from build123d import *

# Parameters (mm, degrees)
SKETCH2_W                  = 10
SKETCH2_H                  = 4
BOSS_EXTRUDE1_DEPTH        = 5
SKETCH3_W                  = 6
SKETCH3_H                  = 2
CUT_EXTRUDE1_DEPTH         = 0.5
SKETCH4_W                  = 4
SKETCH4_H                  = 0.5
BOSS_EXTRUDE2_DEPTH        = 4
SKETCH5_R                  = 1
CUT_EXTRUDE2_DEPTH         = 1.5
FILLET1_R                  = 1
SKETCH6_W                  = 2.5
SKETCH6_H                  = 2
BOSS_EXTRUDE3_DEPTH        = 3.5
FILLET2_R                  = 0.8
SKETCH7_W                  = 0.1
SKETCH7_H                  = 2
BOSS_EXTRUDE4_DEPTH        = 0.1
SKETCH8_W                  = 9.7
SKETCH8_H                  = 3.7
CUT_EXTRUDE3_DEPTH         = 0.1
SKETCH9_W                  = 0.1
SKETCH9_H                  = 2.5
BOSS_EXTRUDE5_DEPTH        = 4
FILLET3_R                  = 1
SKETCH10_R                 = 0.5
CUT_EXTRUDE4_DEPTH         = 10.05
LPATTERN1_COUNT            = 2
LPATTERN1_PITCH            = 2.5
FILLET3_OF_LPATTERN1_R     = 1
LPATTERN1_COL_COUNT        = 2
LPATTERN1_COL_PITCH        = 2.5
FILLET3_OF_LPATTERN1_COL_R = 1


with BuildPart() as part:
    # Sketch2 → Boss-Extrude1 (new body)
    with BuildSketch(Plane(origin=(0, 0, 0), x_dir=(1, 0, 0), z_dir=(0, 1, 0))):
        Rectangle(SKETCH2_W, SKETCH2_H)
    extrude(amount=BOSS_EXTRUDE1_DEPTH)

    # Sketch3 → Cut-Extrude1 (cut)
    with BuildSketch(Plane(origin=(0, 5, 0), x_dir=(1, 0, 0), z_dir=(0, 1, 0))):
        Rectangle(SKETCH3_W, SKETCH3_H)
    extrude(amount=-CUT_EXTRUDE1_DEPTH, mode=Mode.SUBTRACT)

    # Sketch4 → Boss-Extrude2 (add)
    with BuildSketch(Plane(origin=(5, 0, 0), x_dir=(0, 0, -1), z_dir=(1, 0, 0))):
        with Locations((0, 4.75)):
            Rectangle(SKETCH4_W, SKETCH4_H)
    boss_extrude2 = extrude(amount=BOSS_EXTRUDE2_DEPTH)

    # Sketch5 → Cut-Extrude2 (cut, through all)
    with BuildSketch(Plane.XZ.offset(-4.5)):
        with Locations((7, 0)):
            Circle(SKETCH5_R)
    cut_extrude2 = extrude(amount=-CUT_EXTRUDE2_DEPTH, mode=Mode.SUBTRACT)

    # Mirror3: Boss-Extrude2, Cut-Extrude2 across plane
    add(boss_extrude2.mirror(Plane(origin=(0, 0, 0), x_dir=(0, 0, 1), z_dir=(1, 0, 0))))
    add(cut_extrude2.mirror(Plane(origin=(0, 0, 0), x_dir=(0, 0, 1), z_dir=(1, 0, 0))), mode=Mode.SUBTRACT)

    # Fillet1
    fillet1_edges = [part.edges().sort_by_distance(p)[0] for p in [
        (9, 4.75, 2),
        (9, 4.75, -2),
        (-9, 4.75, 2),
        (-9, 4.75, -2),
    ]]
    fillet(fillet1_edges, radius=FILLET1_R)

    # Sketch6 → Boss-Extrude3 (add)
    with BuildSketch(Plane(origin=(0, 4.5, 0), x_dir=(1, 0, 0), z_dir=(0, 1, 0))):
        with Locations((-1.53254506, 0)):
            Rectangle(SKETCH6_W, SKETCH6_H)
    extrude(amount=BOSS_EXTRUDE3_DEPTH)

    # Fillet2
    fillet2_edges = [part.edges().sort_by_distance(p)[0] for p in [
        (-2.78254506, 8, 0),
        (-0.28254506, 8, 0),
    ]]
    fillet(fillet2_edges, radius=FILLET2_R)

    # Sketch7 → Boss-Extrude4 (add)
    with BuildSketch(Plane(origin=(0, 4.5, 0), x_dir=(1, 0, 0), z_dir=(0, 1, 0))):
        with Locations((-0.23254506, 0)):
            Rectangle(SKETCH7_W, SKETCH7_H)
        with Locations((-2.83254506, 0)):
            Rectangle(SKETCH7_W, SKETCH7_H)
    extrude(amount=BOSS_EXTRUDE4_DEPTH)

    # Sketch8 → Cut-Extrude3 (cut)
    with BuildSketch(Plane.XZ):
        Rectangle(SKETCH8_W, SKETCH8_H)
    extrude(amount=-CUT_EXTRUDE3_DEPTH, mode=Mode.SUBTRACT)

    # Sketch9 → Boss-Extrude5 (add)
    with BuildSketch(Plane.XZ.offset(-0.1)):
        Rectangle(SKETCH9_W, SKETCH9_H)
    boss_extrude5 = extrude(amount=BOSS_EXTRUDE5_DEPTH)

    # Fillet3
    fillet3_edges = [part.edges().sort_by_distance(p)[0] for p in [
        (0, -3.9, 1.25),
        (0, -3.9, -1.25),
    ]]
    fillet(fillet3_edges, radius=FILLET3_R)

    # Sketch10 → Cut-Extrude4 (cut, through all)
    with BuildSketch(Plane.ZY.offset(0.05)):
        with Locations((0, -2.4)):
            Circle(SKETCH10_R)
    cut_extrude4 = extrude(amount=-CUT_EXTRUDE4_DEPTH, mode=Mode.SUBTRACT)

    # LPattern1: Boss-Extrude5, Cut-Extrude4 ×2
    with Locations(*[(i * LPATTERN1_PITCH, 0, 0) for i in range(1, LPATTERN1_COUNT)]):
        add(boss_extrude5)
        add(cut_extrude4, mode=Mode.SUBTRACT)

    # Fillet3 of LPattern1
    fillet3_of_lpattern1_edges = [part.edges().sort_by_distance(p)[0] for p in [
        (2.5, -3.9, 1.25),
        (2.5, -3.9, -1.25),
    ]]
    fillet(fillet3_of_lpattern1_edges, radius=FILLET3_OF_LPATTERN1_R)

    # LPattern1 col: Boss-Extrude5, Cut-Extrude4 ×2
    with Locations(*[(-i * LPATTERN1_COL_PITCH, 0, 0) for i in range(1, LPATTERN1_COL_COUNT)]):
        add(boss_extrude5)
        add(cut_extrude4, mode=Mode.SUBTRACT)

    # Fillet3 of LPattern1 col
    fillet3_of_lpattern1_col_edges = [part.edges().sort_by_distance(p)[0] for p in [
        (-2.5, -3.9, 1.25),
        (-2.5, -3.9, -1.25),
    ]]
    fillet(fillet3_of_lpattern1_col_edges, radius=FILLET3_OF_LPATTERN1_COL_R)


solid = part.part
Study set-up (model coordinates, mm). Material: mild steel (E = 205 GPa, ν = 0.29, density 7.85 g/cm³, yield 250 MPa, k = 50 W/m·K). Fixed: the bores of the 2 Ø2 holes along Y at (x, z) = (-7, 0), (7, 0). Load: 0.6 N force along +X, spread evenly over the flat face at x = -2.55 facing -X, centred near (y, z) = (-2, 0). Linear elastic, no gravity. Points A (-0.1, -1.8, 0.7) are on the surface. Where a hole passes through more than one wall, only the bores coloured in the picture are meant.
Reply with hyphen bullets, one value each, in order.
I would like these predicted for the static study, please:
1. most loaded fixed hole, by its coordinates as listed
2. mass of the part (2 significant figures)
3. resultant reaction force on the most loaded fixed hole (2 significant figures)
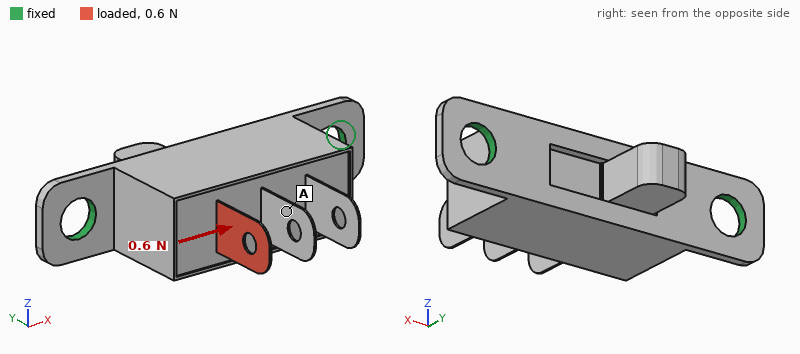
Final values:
- (7, 0)
- 1.7 g
- 0.51 N
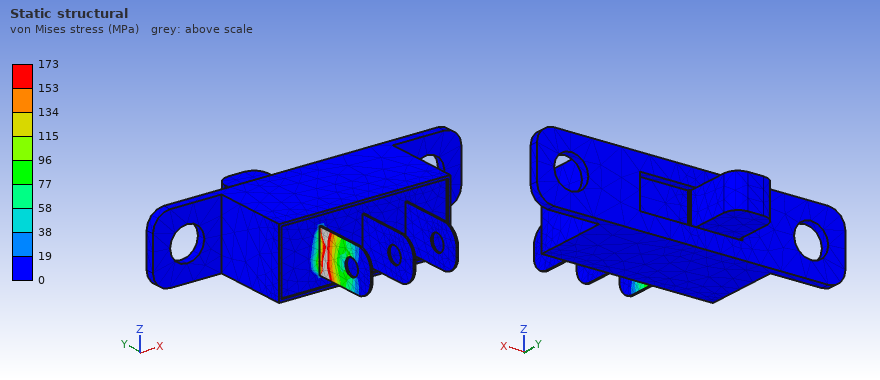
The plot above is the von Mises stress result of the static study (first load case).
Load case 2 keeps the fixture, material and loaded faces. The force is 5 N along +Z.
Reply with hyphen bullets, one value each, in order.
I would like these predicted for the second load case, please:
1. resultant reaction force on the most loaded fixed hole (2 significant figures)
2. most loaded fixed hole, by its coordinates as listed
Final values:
- 3.5 N
- (-7, 0)
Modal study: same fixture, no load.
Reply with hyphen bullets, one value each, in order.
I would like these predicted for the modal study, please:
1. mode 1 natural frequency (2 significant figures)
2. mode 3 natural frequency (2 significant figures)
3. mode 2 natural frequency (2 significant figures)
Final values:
- 5800 Hz
- 5900 Hz
- 5800 Hz
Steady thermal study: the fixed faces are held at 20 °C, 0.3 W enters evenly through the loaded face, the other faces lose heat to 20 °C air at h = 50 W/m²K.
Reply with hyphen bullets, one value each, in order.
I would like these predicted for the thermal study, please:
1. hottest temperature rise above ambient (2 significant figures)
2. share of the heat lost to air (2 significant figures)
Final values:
- 53 K
- 19 %
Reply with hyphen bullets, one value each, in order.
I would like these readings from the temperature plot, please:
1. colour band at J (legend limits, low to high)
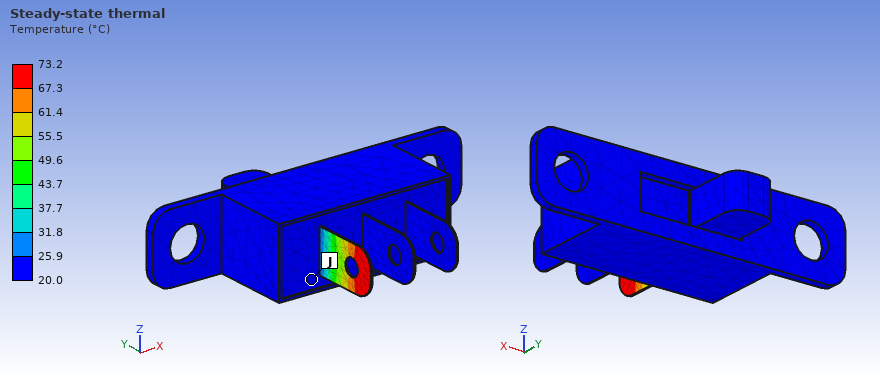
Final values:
- 20.0 to 25.9 °C
